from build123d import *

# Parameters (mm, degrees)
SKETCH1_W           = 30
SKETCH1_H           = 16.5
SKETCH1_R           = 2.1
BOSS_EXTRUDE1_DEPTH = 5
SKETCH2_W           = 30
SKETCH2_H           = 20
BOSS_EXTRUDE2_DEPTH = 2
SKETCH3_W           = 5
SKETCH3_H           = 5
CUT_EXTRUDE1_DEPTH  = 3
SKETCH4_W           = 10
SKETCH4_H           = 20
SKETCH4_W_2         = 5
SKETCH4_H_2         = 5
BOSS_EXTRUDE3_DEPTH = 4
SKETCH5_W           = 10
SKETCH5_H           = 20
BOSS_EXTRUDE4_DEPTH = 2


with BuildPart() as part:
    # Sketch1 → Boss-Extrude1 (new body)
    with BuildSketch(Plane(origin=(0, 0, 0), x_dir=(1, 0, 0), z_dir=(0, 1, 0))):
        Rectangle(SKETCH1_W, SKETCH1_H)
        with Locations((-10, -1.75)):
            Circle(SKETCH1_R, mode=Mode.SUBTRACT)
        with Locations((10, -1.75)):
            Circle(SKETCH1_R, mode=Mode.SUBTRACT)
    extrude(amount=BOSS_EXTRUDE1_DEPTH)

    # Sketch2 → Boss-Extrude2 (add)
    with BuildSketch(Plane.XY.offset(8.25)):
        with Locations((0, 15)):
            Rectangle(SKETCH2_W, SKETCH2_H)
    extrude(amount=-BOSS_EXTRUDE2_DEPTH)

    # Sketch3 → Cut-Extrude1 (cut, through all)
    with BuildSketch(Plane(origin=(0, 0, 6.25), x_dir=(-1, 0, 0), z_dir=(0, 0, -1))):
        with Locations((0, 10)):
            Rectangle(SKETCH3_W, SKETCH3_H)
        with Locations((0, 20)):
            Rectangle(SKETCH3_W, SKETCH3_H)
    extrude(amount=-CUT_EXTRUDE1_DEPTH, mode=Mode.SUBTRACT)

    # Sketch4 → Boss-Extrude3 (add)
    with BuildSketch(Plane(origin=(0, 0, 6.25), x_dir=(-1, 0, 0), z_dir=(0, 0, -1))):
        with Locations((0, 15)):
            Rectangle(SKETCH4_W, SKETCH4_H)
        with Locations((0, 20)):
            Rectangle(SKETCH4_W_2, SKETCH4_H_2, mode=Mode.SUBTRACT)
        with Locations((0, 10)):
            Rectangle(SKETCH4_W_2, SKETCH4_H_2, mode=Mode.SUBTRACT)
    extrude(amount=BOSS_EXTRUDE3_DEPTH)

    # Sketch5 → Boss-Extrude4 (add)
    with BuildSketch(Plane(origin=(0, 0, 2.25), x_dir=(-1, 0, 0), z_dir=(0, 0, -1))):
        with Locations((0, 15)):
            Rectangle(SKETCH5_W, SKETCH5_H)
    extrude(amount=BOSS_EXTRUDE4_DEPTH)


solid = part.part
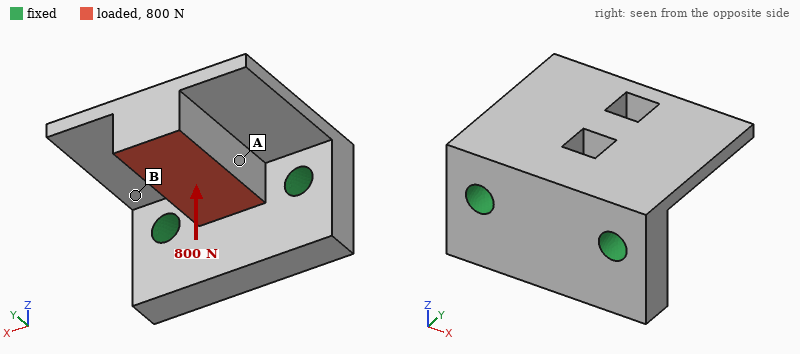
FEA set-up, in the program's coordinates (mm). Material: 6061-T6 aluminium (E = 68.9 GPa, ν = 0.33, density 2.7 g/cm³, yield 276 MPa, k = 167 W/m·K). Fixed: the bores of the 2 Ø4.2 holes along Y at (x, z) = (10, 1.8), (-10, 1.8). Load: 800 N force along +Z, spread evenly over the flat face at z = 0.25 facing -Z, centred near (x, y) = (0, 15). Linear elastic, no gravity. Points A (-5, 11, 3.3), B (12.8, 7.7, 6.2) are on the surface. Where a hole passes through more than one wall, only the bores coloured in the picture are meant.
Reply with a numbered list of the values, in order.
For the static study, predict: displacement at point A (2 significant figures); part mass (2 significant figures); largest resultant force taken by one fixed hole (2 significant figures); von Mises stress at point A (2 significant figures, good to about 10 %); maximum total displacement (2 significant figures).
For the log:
1. 23 µm
2. 12 g
3. 400 N
4. 32 MPa
5. 71 µm
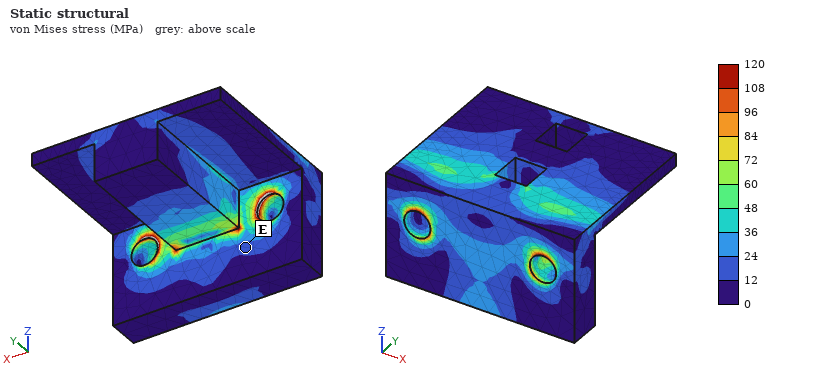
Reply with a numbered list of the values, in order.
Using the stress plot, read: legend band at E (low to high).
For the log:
1. 12 to 24 MPa
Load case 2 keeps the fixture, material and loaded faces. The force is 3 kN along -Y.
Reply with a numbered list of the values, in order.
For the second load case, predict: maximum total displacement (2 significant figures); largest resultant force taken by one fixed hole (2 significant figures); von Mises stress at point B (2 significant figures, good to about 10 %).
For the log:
1. 0.10 mm
2. 1.5 kN
3. 35 MPa
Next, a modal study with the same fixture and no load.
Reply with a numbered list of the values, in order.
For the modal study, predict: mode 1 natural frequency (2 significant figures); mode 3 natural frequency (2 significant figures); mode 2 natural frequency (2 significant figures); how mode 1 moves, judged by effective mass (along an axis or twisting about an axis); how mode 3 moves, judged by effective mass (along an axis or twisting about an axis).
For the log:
1. 8300 Hz
2. 18 kHz
3. 12 kHz
4. along Z
5. along X
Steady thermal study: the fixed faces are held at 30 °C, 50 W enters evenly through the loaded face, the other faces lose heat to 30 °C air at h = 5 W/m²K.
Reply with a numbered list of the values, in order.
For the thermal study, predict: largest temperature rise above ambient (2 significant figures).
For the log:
1. 53 K
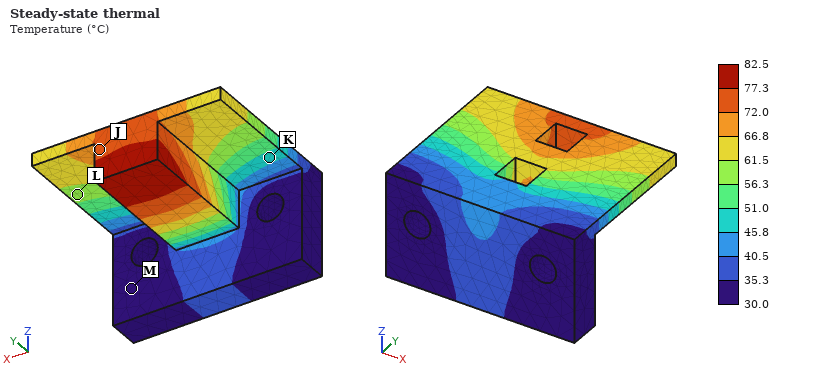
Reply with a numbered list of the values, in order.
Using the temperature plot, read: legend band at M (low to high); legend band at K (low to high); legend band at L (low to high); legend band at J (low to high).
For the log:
1. 30.0 to 35.3 °C
2. 45.8 to 51.0 °C
3. 56.3 to 61.5 °C
4. 72.0 to 77.3 °C
